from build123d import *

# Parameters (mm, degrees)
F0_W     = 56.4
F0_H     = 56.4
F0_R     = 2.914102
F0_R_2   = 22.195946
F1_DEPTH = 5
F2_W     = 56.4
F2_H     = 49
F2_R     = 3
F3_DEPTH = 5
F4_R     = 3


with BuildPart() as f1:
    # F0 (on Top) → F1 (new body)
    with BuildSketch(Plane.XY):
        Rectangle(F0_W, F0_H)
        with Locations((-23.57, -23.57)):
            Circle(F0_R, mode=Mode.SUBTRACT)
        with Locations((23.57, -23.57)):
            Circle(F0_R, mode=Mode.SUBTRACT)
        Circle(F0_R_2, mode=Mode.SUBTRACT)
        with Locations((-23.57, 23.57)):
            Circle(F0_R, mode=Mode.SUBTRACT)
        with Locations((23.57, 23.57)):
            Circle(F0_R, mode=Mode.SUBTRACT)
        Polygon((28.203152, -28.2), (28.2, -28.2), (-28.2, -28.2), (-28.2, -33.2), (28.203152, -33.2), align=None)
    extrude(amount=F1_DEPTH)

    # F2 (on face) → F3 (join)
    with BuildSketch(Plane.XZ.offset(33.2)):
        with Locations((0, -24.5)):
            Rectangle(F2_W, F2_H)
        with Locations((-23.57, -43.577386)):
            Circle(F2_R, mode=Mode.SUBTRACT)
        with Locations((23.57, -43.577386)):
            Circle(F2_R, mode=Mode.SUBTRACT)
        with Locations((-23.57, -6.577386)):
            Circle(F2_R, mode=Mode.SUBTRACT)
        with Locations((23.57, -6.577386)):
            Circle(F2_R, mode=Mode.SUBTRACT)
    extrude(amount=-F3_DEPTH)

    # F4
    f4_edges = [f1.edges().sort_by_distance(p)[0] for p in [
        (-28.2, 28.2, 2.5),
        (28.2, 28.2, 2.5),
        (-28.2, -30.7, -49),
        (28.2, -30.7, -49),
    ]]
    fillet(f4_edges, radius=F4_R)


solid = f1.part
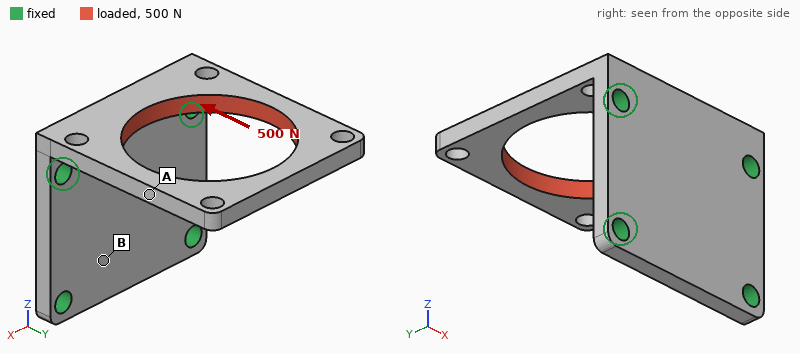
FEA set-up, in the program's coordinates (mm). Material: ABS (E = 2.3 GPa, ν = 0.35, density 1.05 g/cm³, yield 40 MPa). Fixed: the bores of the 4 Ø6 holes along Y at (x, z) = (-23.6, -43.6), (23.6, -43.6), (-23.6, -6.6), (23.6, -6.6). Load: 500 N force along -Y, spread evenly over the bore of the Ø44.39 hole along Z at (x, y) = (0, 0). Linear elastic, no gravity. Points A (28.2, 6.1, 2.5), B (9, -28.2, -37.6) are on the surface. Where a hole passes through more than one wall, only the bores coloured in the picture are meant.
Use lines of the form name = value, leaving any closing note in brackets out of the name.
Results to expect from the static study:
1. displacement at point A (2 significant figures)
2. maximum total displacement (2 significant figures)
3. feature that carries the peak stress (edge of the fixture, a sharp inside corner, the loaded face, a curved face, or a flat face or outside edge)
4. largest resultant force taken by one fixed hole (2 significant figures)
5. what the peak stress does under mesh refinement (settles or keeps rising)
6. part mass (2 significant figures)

displacement at point A = 0.62 mm
maximum total displacement = 1.0 mm
feature that carries the peak stress = edge of the fixture
largest resultant force taken by one fixed hole = 260 N
what the peak stress does under mesh refinement = keeps rising
part mass = 23 g
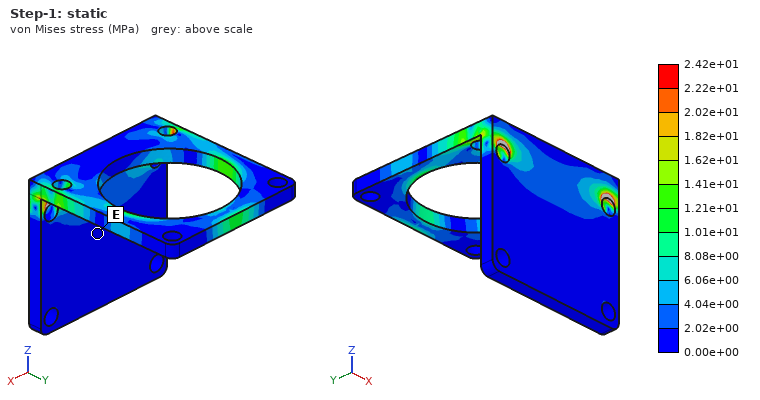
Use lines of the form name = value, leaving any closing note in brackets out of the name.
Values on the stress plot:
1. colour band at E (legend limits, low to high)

colour band at E = 0.00e+00 to 2.02e+00 MPa
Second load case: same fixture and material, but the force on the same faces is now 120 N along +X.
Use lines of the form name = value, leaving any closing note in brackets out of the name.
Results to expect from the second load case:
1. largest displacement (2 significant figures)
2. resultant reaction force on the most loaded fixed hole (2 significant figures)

largest displacement = 0.51 mm
resultant reaction force on the most loaded fixed hole = 96 N
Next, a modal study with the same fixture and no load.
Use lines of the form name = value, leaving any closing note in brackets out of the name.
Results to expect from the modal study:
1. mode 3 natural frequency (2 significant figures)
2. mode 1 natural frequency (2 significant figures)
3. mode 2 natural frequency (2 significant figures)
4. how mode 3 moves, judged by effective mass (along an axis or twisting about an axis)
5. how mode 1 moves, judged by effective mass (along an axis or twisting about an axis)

mode 3 natural frequency = 970 Hz
mode 1 natural frequency = 250 Hz
mode 2 natural frequency = 590 Hz
how mode 3 moves, judged by effective mass = along X
how mode 1 moves, judged by effective mass = along Z
